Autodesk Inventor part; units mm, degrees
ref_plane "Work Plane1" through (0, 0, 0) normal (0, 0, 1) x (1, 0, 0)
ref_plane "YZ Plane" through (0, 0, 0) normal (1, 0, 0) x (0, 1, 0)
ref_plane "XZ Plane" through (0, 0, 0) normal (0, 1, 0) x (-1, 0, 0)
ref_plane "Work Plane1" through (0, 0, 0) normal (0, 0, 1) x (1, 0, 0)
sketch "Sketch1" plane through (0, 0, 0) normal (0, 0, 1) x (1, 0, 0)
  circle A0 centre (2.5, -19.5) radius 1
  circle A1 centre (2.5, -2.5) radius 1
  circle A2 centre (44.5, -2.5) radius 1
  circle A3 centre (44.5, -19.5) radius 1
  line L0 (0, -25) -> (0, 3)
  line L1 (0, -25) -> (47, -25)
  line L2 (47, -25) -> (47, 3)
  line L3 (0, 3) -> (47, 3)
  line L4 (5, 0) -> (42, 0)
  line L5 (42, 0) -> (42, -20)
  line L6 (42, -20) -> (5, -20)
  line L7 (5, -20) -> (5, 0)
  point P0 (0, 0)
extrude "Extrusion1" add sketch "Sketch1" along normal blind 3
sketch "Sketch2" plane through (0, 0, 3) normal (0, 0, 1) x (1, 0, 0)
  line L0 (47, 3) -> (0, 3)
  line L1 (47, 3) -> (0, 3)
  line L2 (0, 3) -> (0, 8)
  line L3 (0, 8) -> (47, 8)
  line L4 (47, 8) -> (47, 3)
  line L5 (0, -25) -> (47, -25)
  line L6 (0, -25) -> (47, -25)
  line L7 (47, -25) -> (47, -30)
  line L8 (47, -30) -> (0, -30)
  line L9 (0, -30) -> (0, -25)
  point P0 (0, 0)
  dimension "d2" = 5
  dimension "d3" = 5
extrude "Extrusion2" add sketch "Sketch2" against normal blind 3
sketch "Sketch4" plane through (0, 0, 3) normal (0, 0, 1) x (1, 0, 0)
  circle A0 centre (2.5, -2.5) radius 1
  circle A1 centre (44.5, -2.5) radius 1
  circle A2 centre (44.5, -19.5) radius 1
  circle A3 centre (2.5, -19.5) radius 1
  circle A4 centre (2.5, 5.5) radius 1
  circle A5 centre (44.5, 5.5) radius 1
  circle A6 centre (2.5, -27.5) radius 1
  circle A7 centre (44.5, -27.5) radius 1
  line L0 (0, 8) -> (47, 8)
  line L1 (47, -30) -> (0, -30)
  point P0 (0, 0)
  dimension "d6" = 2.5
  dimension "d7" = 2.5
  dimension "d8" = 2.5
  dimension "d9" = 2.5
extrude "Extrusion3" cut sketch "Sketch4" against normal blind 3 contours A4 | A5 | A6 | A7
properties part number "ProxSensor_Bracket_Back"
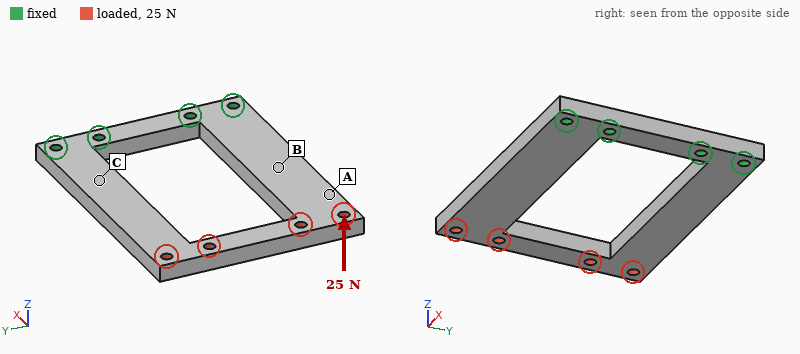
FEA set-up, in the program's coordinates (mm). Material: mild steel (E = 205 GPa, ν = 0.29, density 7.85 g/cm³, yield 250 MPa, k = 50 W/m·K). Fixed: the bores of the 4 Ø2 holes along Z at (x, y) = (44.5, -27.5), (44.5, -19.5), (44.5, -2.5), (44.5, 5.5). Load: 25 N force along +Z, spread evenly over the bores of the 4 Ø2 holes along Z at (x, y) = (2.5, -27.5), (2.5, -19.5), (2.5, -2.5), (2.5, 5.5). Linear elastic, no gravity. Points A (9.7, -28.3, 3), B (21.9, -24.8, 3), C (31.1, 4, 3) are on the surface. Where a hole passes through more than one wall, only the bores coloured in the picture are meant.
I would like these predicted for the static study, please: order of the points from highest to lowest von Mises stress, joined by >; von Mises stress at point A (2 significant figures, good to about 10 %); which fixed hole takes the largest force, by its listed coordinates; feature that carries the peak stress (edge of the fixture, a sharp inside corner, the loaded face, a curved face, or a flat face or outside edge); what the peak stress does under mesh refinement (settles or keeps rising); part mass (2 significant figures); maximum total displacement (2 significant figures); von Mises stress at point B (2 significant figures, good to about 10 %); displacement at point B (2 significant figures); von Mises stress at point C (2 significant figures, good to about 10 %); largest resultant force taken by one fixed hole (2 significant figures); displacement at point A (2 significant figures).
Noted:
C > B > A
6.8 MPa
(44.5, 5.5)
edge of the fixture
keeps rising
24 g
81 µm
18 MPa
26 µm
27 MPa
14 N
54 µm
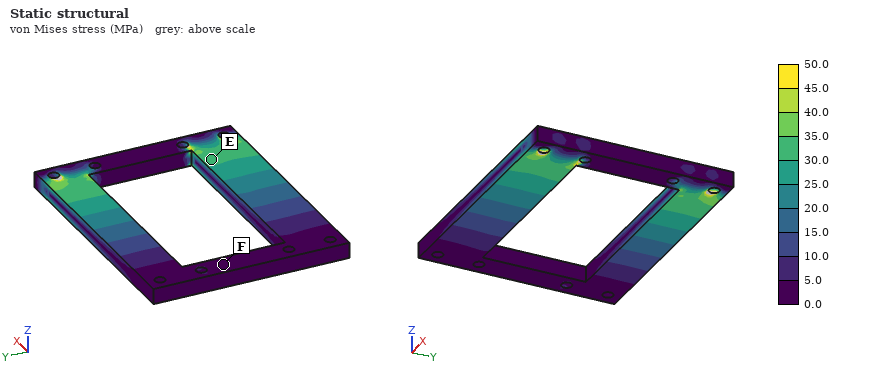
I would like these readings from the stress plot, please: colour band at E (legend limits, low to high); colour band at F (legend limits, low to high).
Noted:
30.0 to 35.0 MPa
0.0 to 5.0 MPa
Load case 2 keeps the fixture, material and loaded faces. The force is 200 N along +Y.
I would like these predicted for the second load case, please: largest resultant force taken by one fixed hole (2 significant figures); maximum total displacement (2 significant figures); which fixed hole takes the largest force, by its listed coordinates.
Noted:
480 N
37 µm
(44.5, -27.5)
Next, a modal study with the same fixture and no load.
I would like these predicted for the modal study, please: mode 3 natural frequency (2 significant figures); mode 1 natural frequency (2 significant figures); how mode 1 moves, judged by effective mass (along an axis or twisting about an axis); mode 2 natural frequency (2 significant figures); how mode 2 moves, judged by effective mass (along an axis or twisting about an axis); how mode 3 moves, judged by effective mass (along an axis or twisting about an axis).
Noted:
4200 Hz
1100 Hz
along Z
2500 Hz
twisting about X
along Y
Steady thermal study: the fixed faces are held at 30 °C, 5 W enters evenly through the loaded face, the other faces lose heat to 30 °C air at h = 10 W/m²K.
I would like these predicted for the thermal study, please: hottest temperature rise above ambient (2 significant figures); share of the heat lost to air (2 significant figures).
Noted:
72 K
19 %
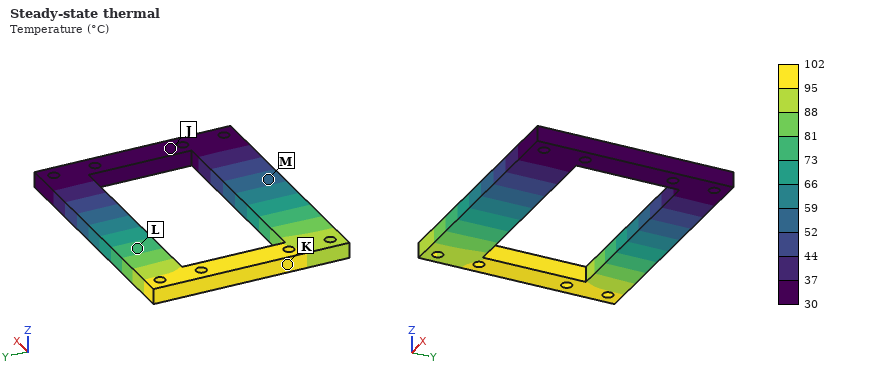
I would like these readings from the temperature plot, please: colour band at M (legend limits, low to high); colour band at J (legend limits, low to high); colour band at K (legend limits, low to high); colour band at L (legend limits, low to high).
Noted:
52 to 59 °C
30 to 37 °C
95 to 102 °C
73 to 81 °C
